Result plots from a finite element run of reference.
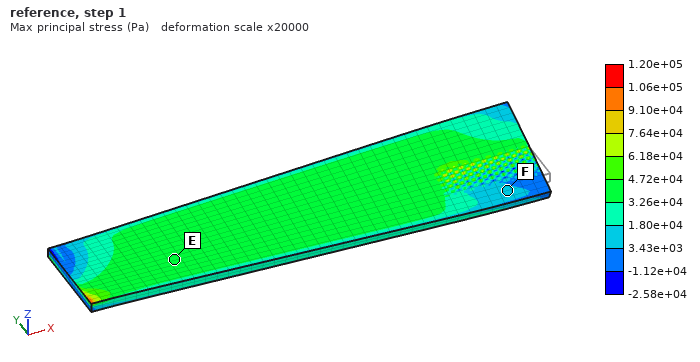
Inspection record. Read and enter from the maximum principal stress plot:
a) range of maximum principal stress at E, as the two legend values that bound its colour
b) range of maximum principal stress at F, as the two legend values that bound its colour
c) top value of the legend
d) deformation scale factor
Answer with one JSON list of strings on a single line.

["3.26e+04 to 4.72e+04 Pa", "3.43e+03 to 1.80e+04 Pa", "1.20e+05 Pa", "20000"]
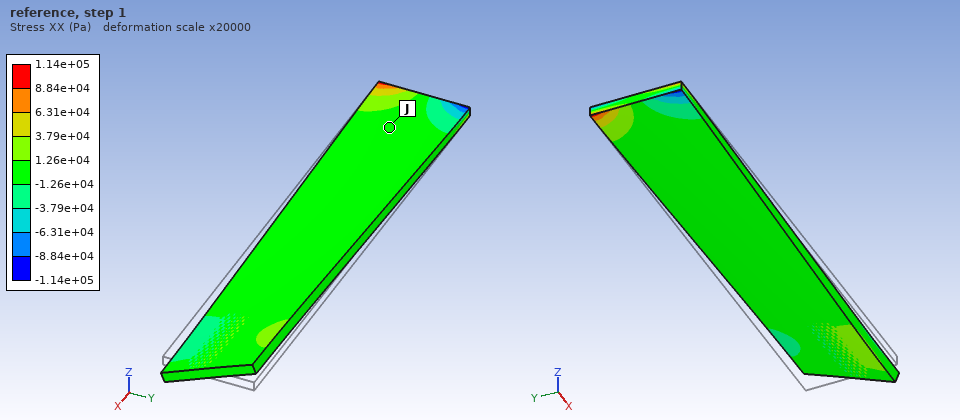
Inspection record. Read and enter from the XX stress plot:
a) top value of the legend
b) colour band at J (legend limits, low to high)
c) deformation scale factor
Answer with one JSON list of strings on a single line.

["1.14e+05 Pa", "-1.26e+04 to 1.26e+04 Pa", "20000"]
